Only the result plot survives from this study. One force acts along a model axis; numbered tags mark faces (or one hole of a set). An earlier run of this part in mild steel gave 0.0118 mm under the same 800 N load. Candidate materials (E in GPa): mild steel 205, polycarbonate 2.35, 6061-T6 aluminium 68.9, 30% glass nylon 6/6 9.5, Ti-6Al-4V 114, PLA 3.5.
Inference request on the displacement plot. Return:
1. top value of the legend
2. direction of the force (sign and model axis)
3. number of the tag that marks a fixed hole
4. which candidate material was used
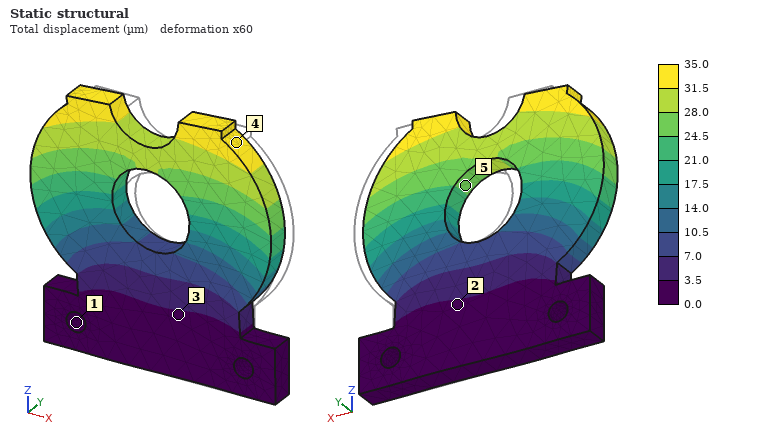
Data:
35.0 µm
-X
1
6061-T6 aluminium
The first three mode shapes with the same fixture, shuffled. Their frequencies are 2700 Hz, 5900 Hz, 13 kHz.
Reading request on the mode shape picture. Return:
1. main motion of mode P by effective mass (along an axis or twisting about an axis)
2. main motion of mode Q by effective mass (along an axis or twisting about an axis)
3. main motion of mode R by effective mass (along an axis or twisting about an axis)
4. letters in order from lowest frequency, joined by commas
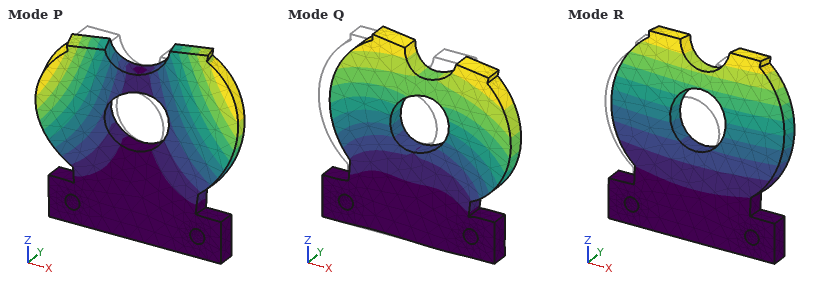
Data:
twisting about Z
along X
along Y
R, P, Q
